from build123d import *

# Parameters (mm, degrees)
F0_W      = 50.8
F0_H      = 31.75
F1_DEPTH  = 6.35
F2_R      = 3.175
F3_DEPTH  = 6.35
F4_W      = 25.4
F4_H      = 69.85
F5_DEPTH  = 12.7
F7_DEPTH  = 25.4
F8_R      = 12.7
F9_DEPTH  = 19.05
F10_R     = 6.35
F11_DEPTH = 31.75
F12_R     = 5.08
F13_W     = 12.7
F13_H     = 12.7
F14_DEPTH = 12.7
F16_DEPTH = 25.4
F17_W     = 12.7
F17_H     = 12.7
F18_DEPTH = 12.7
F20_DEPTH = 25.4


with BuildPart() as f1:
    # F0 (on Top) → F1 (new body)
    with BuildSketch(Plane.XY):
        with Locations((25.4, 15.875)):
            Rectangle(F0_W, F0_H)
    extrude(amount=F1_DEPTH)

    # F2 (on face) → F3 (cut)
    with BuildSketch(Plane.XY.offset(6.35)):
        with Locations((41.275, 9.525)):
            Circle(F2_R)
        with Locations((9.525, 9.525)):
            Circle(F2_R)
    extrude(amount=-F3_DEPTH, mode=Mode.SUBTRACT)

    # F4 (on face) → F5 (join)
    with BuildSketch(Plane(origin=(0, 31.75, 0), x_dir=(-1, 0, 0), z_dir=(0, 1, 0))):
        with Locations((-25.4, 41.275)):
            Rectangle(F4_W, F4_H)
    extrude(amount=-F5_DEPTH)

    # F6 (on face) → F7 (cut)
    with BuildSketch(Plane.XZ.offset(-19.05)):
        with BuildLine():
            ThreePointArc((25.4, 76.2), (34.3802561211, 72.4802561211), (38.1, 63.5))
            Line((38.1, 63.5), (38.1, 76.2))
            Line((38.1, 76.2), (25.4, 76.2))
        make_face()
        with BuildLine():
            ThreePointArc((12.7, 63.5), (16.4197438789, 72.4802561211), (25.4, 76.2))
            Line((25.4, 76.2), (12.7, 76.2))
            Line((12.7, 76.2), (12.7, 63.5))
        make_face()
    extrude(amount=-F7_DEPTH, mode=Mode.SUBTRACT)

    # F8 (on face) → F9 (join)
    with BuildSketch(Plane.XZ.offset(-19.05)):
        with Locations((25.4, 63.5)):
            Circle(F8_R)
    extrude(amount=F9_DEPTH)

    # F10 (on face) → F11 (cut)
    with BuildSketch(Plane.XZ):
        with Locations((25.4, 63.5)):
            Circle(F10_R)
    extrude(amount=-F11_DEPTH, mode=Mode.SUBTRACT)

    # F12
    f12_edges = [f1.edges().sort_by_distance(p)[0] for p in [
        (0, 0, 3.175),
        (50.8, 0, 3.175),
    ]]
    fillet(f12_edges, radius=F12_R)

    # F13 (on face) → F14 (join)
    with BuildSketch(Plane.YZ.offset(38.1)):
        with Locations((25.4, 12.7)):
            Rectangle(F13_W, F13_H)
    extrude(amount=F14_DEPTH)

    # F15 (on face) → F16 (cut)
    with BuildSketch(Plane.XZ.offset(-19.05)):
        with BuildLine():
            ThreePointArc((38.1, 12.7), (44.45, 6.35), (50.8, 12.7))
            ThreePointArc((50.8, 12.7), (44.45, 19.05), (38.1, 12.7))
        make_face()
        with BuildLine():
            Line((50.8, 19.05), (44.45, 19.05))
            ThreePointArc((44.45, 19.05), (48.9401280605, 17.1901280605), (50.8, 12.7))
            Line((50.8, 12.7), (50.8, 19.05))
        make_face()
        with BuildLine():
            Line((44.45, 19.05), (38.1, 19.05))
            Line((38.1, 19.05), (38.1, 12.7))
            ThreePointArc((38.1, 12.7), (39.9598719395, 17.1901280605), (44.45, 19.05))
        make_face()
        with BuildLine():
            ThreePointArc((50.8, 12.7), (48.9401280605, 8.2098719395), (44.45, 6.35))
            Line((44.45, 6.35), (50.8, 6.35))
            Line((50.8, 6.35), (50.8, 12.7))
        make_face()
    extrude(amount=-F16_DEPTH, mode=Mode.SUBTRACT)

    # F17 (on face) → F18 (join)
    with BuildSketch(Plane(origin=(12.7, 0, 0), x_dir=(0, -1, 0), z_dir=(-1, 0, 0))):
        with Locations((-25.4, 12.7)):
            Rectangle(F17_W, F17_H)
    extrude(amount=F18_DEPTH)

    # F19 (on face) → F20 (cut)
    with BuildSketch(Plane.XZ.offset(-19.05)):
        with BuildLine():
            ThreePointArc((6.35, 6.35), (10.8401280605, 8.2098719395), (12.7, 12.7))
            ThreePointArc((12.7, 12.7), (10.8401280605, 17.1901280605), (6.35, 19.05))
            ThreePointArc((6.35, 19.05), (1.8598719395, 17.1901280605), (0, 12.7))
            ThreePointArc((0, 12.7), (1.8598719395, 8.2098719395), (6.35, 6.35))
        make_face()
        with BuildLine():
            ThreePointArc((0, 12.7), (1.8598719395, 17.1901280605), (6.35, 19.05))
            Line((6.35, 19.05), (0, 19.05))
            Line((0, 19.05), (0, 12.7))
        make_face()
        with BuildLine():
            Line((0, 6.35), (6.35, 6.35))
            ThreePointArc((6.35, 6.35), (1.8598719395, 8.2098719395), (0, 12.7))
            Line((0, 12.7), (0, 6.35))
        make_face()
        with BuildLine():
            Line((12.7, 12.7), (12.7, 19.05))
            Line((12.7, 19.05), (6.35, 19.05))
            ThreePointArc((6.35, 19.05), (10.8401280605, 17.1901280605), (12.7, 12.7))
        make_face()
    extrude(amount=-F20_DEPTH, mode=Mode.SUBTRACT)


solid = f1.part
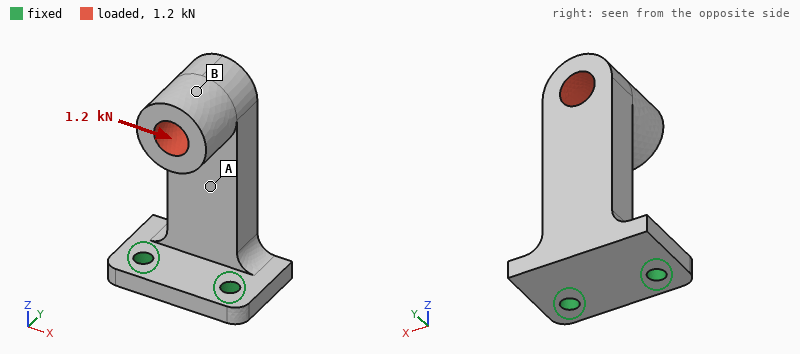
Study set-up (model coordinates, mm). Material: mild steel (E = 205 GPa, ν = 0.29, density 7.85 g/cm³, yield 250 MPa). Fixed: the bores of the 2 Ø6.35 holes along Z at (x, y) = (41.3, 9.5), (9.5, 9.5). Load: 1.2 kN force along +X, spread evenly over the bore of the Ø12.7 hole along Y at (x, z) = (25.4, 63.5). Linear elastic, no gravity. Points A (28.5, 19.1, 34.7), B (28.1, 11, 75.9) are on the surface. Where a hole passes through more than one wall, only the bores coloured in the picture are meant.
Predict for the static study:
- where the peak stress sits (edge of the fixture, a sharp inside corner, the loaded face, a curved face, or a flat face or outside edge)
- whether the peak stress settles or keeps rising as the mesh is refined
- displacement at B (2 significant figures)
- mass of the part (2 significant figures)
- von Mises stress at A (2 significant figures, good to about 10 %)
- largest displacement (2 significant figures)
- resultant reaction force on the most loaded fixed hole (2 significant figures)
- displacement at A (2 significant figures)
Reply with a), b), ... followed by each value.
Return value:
a) edge of the fixture
b) keeps rising
c) 0.097 mm
d) 290 g
e) 30 MPa
f) 0.11 mm
g) 2.3 kN
h) 0.034 mm
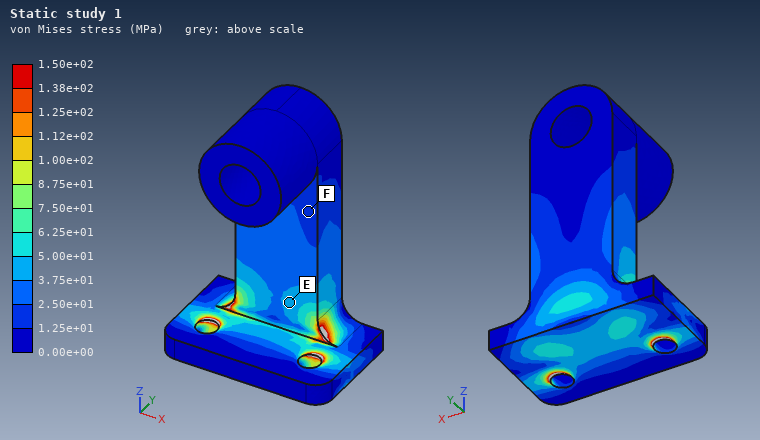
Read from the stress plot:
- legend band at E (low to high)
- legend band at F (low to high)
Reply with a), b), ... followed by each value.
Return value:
a) 3.75e+01 to 5.00e+01 MPa
b) 1.25e+01 to 2.50e+01 MPa
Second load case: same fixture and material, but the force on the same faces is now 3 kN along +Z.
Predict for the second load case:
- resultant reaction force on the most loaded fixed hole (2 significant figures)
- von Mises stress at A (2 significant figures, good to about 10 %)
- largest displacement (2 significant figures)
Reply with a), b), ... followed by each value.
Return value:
a) 1.5 kN
b) 51 MPa
c) 96 µm
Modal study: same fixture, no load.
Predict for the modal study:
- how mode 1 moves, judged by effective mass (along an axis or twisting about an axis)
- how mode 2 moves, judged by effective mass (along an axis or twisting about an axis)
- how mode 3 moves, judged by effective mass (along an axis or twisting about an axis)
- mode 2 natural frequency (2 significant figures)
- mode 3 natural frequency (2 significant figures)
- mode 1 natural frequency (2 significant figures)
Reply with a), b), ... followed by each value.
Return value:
a) along Y
b) along X
c) along Z
d) 1800 Hz
e) 4400 Hz
f) 830 Hz
